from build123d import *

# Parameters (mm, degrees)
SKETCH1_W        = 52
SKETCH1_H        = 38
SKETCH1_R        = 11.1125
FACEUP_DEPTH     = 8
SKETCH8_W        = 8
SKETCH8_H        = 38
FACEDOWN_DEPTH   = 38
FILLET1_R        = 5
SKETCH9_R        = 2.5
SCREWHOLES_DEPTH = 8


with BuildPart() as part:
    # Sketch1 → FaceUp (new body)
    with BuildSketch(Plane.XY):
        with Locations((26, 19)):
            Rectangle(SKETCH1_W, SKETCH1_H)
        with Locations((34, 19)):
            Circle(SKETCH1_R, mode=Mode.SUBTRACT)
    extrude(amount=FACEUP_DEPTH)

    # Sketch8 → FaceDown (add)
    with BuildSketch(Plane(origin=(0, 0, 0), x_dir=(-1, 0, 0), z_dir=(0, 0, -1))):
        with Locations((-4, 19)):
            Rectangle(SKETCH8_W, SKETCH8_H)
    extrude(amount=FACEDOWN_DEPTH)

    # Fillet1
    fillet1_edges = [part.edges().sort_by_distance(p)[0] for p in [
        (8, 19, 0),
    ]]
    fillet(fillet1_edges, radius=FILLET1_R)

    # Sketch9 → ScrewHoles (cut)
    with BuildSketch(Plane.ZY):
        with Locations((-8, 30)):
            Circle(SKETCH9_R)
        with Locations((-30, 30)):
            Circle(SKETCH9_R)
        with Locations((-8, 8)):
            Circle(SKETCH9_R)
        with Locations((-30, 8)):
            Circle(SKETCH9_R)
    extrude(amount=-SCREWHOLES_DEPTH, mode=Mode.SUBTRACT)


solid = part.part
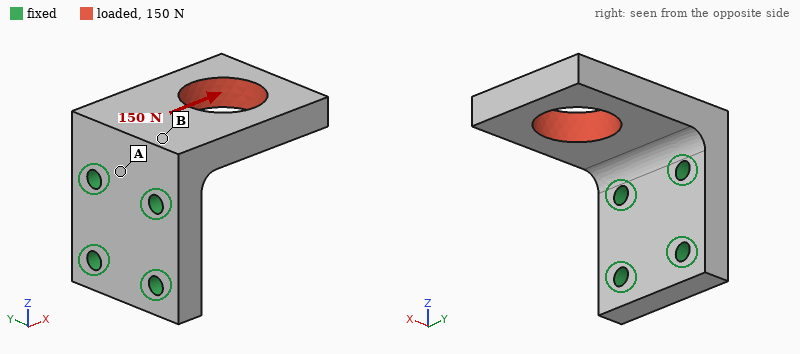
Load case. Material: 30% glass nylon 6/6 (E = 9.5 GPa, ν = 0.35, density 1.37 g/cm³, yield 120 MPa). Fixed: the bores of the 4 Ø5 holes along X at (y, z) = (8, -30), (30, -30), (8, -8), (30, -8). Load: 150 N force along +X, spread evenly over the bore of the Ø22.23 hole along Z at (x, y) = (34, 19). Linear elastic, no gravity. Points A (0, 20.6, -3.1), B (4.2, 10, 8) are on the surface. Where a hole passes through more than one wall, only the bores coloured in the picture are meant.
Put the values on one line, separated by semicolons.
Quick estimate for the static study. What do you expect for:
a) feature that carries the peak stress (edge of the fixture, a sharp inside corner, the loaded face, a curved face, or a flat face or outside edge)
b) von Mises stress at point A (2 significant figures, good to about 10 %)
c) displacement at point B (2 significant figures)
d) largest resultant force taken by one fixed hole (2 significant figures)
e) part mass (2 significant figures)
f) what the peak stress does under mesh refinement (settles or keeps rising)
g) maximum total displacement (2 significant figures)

edge of the fixture; 1.4 MPa; 9.3 µm; 83 N; 33 g; keeps rising; 35 µm
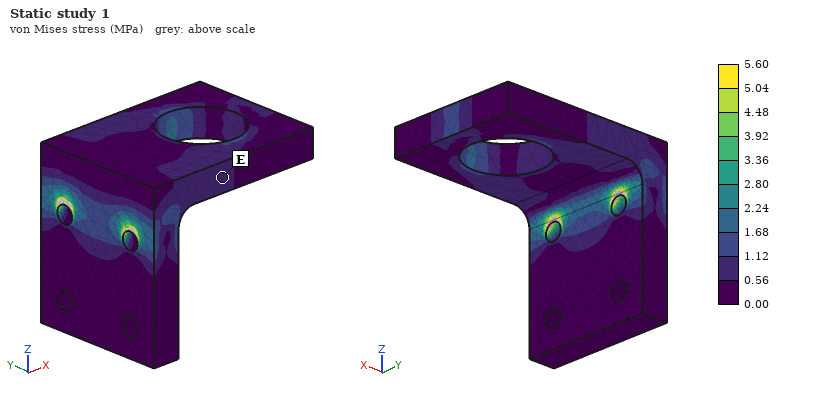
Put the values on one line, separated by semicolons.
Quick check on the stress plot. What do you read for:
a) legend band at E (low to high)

0.56 to 1.12 MPa
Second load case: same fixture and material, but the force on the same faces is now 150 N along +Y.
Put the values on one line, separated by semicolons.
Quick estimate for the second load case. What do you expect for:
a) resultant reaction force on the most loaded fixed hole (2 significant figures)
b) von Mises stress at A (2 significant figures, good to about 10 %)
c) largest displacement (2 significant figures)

190 N; 1.5 MPa; 59 µm
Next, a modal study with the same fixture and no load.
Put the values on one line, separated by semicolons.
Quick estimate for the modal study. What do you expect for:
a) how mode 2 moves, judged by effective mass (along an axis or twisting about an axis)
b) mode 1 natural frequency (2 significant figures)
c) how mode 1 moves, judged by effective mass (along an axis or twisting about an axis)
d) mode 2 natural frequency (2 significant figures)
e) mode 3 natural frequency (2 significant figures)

along Y; 1300 Hz; along Z; 2700 Hz; 3500 Hz
